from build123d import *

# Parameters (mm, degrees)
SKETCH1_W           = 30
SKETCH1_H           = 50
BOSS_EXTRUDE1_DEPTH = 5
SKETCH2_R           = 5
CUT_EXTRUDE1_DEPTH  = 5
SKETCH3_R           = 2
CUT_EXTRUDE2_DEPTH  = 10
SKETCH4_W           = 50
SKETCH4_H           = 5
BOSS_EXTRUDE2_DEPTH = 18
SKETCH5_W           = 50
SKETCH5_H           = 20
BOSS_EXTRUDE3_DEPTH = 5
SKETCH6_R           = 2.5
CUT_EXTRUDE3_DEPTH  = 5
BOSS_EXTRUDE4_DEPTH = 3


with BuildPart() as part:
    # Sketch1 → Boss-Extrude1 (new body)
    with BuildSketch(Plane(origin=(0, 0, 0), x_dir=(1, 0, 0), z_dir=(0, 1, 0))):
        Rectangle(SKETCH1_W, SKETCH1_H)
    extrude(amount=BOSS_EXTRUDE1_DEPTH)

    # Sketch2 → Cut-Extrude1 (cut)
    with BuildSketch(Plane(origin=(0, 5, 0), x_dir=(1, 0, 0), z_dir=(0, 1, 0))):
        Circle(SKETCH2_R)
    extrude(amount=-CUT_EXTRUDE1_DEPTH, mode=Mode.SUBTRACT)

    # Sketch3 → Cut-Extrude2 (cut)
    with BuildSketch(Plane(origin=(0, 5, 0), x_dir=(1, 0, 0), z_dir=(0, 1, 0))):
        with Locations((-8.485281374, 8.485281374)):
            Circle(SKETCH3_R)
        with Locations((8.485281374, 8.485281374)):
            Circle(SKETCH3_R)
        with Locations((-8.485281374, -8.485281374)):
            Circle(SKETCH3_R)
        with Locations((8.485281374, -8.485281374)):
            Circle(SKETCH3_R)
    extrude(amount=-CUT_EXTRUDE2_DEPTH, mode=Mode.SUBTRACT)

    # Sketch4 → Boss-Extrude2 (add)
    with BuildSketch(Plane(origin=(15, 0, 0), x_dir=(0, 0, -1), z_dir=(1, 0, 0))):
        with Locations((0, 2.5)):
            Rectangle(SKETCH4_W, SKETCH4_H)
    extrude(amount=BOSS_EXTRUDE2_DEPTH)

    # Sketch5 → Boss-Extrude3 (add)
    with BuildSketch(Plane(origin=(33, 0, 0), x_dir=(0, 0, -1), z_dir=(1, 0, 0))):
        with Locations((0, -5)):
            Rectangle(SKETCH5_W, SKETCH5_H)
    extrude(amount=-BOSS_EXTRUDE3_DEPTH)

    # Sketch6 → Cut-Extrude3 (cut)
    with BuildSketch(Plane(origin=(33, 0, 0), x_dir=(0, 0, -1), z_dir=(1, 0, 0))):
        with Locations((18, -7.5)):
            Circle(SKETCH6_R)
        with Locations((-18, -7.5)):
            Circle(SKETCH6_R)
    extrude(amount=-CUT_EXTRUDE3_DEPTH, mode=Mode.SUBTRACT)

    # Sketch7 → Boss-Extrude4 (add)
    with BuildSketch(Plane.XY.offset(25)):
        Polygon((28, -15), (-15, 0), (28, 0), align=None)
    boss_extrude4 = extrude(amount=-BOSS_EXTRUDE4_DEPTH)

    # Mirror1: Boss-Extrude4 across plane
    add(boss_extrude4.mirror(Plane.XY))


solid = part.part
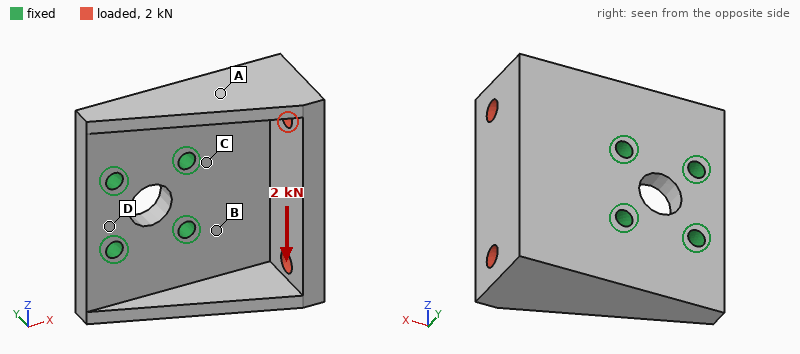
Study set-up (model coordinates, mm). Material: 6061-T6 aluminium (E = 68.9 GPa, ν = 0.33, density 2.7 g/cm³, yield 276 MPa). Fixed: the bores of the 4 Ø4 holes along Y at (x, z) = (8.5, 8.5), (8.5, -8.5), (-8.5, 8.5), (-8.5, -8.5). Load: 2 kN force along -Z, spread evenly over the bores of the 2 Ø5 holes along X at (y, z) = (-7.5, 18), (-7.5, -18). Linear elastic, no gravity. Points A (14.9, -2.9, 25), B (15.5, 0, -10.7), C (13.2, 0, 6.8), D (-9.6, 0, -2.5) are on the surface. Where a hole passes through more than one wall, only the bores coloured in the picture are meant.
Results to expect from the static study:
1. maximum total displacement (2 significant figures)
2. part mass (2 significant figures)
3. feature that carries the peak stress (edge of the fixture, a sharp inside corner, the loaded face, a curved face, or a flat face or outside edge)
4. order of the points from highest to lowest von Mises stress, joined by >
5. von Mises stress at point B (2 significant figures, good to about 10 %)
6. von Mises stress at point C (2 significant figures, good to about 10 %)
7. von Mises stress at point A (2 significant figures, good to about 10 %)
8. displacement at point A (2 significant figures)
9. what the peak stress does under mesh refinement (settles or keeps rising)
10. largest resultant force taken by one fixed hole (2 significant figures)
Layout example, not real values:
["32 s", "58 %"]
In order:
["0.12 mm", "45 g", "edge of the fixture", "C > B > A > D", "52 MPa", "64 MPa", "25 MPa", "0.050 mm", "keeps rising", "2.0 kN"]
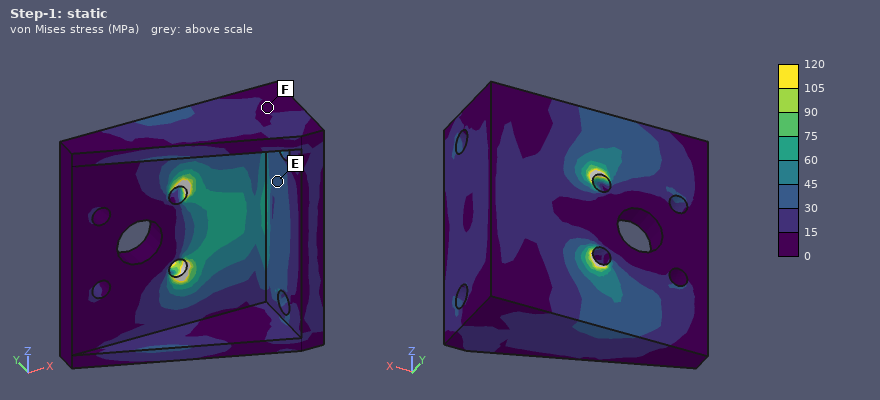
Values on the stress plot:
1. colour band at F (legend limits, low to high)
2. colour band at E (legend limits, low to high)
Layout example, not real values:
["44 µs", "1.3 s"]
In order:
["0 to 15 MPa", "30 to 45 MPa"]
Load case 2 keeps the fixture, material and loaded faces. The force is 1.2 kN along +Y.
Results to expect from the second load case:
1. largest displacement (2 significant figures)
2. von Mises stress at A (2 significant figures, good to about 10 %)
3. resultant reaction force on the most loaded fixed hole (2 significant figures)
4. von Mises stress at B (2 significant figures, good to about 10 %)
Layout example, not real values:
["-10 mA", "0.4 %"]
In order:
["0.11 mm", "18 MPa", "970 N", "50 MPa"]
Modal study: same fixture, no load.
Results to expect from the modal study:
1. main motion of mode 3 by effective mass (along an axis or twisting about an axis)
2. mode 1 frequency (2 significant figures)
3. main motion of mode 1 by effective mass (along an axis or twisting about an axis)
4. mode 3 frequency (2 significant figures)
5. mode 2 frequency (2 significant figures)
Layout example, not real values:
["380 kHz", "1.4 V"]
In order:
["along Y", "4300 Hz", "along Y", "11 kHz", "4700 Hz"]
